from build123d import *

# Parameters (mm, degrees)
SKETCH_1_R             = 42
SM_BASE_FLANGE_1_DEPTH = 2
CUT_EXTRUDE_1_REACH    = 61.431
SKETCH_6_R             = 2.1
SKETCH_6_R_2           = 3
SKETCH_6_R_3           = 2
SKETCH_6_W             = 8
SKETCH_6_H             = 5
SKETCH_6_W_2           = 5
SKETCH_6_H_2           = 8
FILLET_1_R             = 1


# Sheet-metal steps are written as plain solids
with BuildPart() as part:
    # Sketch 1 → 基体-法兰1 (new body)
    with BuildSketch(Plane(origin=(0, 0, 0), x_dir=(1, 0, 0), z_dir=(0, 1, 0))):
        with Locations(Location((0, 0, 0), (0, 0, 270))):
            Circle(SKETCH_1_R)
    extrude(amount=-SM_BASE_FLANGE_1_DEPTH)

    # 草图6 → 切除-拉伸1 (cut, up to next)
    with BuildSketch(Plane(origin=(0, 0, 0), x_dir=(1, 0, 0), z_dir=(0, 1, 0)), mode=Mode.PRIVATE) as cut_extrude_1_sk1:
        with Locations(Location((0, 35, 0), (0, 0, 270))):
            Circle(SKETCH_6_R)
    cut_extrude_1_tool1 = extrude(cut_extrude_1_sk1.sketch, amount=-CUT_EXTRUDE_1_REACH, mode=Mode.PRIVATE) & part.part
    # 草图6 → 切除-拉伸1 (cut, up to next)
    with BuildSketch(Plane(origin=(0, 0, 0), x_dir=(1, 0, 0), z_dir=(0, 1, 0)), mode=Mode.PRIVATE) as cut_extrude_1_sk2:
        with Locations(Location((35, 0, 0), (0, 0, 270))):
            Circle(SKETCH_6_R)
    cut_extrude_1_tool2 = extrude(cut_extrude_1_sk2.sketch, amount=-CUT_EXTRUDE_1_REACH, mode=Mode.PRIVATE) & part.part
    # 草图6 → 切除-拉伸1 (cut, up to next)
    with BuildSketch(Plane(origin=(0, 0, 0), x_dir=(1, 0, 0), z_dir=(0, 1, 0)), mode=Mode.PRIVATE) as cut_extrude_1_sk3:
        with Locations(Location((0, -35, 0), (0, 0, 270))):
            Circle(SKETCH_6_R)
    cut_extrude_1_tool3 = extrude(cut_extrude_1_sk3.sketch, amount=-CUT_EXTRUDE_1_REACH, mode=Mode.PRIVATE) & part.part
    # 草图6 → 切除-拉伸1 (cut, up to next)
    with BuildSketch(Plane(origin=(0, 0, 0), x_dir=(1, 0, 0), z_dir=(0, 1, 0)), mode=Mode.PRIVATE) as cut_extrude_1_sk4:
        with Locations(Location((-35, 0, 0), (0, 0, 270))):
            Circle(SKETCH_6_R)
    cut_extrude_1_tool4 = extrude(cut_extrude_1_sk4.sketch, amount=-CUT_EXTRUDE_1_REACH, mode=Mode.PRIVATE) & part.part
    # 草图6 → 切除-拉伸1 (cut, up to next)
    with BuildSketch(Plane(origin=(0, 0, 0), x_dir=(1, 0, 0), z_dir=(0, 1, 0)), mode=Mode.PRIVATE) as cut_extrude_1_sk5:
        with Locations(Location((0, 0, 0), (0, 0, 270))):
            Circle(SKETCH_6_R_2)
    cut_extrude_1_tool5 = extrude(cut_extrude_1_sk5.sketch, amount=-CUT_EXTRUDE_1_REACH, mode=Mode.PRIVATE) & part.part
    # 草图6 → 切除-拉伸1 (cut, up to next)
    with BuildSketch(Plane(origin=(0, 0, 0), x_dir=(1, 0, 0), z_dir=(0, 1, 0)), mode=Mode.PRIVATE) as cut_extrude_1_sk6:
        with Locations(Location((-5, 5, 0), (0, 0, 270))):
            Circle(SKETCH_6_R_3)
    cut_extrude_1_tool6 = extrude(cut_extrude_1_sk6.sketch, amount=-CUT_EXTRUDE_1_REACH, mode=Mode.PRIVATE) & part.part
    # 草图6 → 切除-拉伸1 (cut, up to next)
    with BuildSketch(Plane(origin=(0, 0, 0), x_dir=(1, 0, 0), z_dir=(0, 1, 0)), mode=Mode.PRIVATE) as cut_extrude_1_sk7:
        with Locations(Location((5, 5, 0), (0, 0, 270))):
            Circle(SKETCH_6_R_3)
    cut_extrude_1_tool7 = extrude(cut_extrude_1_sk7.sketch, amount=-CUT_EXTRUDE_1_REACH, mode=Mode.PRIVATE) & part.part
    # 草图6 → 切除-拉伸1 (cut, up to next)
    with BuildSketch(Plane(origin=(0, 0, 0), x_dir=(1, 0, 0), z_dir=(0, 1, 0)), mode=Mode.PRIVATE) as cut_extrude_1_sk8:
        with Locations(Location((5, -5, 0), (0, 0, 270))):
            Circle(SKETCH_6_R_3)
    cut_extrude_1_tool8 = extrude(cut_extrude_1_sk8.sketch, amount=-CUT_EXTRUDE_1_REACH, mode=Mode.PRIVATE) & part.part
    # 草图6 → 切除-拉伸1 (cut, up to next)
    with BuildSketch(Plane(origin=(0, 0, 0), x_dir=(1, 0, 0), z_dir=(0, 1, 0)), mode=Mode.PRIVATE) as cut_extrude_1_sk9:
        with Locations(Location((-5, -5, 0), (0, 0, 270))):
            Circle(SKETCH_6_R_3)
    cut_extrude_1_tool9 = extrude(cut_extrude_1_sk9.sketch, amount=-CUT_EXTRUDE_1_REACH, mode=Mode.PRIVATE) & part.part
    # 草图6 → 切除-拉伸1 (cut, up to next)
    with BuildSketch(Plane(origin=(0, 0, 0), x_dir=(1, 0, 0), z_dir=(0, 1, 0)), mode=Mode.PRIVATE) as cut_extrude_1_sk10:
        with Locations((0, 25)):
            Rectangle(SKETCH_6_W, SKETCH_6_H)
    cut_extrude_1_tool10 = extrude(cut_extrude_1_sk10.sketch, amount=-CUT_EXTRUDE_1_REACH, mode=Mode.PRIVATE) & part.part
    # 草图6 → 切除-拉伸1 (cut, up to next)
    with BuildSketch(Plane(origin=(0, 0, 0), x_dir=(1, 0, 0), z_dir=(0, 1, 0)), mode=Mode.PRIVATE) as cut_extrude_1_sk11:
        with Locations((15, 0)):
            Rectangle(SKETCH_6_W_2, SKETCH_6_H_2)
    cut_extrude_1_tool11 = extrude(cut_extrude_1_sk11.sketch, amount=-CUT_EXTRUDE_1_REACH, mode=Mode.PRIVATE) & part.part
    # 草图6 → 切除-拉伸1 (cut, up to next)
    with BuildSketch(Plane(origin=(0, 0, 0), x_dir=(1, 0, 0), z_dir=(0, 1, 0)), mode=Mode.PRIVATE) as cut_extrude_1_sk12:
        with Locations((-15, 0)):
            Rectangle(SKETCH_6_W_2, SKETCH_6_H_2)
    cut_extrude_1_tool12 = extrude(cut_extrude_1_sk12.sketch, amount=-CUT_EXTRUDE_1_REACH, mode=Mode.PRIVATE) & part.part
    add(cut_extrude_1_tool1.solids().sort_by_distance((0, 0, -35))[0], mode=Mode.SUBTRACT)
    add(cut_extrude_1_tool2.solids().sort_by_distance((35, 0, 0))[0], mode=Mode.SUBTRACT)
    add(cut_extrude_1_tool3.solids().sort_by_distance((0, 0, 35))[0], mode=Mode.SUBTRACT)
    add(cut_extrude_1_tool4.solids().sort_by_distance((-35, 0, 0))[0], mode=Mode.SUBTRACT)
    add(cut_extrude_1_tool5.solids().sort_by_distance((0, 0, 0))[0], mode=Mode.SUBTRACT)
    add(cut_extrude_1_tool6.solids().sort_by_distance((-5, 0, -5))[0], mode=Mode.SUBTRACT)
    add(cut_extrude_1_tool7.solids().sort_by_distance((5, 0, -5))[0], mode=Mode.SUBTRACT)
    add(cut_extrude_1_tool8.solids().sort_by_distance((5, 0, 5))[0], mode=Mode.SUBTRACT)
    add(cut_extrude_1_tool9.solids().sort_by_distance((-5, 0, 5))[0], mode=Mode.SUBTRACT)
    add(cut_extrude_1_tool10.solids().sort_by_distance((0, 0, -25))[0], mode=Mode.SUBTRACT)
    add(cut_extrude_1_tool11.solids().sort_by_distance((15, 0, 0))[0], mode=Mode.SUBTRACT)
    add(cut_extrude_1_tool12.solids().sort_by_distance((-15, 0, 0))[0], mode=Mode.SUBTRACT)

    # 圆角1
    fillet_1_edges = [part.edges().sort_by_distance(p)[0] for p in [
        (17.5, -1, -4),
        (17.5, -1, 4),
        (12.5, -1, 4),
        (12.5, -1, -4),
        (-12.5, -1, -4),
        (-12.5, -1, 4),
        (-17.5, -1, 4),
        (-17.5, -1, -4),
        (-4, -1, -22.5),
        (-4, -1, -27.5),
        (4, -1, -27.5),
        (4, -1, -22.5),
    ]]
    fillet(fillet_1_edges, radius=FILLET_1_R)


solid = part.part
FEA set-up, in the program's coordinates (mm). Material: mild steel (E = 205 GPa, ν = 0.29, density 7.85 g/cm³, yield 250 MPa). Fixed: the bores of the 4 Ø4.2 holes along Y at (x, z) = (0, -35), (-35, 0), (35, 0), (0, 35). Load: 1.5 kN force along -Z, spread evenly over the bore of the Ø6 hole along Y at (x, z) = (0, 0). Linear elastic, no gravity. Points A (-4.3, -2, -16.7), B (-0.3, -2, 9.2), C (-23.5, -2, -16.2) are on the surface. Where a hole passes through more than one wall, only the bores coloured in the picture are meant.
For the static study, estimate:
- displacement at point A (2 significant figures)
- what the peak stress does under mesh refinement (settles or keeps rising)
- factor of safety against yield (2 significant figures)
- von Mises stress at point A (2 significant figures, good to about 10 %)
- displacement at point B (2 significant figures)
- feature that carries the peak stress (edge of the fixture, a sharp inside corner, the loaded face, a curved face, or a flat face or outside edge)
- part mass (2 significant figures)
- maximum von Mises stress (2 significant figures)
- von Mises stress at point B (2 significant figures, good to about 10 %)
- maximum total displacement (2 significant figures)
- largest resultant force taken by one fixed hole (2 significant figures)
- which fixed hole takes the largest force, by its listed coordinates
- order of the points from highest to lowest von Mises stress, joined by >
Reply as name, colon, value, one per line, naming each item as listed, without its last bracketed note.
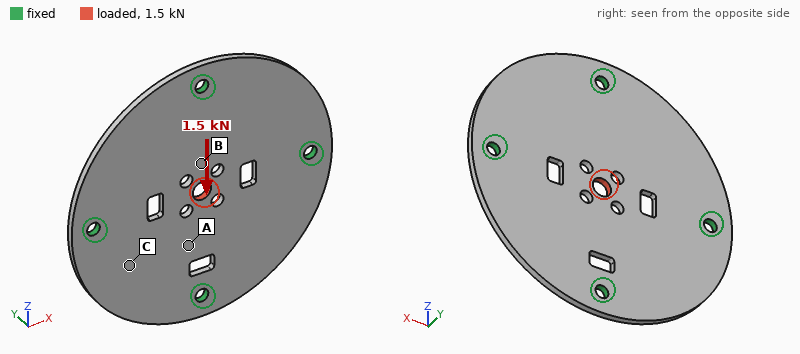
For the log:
displacement at point A: 1.9 µm
what the peak stress does under mesh refinement: settles
factor of safety against yield: 3.0
von Mises stress at point A: 17 MPa
displacement at point B: 2.5 µm
feature that carries the peak stress: a curved face
part mass: 83 g
maximum von Mises stress: 84 MPa
von Mises stress at point B: 31 MPa
maximum total displacement: 4.2 µm
largest resultant force taken by one fixed hole: 530 N
which fixed hole takes the largest force, by its listed coordinates: (0, 35)
order of the points from highest to lowest von Mises stress, joined by >: B > A > C
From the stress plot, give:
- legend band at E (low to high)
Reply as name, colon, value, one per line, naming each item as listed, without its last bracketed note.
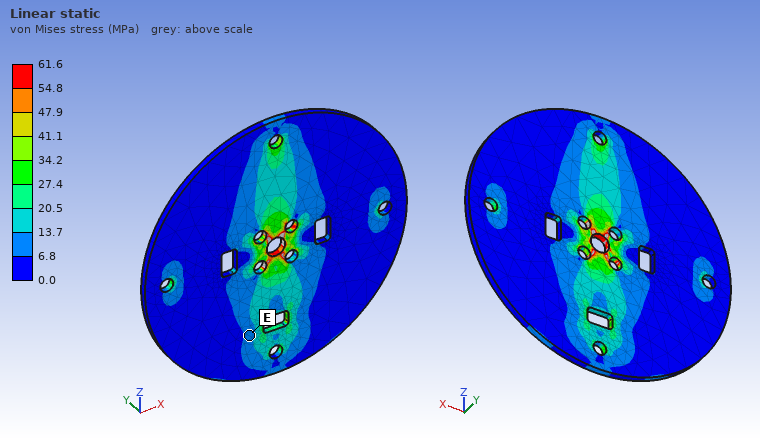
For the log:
legend band at E: 6.8 to 13.7 MPa
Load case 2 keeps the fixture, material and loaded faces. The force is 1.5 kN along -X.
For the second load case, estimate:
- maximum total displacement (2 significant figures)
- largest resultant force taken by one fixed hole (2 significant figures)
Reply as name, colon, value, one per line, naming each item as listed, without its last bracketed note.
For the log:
maximum total displacement: 4.6 µm
largest resultant force taken by one fixed hole: 460 N
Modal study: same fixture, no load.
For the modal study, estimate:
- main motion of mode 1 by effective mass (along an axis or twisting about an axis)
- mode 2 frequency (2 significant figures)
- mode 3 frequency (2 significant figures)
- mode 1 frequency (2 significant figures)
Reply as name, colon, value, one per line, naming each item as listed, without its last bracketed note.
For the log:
main motion of mode 1 by effective mass: along Y
mode 2 frequency: 3500 Hz
mode 3 frequency: 3600 Hz
mode 1 frequency: 3200 Hz
